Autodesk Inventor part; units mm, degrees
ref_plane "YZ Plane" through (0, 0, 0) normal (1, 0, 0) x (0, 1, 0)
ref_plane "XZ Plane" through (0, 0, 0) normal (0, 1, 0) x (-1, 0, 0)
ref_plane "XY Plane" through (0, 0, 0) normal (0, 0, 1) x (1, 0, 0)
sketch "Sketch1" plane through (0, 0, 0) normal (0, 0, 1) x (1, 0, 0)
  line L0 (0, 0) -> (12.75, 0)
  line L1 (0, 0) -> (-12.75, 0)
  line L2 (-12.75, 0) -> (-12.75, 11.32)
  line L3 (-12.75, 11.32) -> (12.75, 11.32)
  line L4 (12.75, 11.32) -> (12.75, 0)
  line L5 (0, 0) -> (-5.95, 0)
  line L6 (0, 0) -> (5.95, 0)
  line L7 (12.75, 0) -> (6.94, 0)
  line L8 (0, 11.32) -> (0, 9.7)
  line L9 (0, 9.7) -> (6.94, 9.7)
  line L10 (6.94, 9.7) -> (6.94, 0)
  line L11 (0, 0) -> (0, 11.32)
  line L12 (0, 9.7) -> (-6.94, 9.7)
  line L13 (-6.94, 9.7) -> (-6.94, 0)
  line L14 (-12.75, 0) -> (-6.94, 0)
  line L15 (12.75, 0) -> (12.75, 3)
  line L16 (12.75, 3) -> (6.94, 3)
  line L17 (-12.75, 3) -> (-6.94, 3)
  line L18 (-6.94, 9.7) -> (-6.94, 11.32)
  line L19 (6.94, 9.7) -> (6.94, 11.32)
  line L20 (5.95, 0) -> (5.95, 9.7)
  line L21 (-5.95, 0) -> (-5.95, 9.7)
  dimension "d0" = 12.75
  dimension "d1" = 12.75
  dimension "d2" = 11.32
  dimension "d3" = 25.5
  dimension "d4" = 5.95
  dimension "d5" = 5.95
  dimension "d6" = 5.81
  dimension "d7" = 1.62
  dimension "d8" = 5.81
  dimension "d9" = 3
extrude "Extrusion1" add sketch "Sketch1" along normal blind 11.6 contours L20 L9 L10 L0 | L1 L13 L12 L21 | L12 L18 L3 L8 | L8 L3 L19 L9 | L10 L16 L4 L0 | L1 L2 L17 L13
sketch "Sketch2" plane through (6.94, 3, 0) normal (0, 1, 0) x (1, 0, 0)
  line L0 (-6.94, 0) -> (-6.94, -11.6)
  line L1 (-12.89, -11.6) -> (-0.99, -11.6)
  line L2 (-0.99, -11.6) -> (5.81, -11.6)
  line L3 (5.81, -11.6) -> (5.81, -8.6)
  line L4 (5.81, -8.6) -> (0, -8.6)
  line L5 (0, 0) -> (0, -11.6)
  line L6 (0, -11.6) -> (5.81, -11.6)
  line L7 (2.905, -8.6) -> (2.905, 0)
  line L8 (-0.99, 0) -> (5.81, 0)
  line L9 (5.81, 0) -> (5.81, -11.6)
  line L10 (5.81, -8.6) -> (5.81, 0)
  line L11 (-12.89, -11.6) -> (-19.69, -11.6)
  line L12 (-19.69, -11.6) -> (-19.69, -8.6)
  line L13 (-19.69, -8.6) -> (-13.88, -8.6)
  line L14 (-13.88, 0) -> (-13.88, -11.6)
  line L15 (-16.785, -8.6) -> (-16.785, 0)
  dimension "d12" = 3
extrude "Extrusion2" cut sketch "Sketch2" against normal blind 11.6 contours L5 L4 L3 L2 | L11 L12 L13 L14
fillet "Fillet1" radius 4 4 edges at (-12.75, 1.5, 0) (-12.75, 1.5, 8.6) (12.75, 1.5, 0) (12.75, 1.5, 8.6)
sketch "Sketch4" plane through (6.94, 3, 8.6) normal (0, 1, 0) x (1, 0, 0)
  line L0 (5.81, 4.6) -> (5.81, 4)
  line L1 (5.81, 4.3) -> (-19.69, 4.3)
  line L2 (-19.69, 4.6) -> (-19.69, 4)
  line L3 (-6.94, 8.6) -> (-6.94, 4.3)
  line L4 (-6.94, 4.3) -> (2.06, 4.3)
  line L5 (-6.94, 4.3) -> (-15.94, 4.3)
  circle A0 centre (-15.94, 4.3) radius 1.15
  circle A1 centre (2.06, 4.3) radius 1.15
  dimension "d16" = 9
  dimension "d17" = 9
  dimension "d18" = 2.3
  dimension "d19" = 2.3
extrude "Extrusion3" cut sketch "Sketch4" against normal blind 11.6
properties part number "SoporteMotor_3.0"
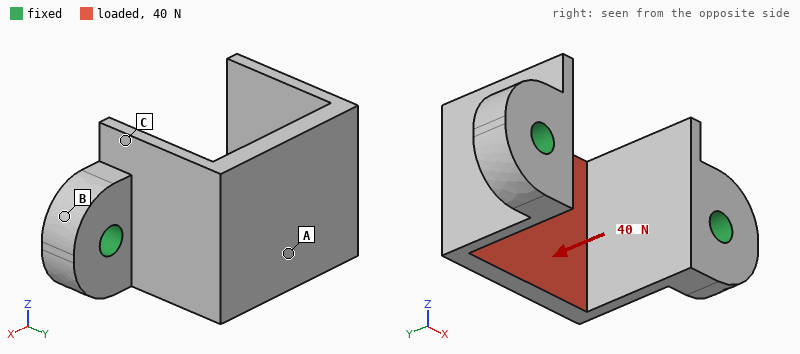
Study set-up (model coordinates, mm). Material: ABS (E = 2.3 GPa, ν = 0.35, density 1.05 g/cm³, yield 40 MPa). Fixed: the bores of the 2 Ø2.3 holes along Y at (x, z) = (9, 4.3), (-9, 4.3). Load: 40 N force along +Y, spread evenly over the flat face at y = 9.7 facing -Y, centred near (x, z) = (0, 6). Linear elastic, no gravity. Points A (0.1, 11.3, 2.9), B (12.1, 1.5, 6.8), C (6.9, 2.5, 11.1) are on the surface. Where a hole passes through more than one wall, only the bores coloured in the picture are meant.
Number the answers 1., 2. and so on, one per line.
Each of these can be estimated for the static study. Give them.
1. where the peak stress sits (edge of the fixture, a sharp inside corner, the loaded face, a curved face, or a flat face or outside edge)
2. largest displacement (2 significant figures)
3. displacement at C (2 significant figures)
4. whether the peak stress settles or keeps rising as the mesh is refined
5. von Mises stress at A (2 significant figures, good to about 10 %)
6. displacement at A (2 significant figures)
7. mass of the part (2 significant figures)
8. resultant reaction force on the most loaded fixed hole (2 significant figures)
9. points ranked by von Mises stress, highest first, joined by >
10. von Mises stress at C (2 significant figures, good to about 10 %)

1. edge of the fixture
2. 0.11 mm
3. 0.021 mm
4. keeps rising
5. 8.6 MPa
6. 0.083 mm
7. 0.75 g
8. 20 N
9. A > C > B
10. 2.2 MPa
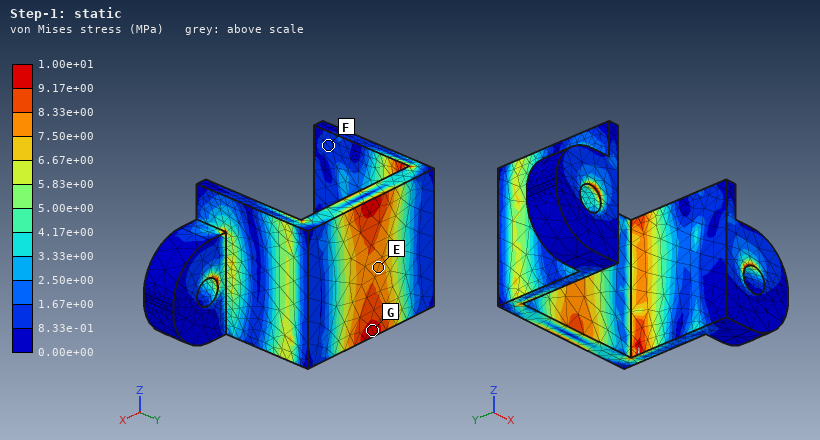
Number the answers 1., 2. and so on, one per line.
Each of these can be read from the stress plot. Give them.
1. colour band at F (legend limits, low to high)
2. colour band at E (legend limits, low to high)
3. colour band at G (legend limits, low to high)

1. 8.33e-01 to 1.67e+00 MPa
2. 7.50e+00 to 8.33e+00 MPa
3. 9.17e+00 to 1.00e+01 MPa
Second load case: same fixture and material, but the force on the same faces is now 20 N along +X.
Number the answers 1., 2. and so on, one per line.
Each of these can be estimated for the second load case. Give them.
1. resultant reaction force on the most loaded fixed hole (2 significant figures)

1. 11 N
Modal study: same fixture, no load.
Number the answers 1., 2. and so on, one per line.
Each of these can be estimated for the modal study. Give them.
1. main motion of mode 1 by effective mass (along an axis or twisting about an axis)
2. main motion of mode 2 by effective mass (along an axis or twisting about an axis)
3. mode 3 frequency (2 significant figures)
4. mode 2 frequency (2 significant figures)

1. along X
2. along Z
3. 6100 Hz
4. 4700 Hz
